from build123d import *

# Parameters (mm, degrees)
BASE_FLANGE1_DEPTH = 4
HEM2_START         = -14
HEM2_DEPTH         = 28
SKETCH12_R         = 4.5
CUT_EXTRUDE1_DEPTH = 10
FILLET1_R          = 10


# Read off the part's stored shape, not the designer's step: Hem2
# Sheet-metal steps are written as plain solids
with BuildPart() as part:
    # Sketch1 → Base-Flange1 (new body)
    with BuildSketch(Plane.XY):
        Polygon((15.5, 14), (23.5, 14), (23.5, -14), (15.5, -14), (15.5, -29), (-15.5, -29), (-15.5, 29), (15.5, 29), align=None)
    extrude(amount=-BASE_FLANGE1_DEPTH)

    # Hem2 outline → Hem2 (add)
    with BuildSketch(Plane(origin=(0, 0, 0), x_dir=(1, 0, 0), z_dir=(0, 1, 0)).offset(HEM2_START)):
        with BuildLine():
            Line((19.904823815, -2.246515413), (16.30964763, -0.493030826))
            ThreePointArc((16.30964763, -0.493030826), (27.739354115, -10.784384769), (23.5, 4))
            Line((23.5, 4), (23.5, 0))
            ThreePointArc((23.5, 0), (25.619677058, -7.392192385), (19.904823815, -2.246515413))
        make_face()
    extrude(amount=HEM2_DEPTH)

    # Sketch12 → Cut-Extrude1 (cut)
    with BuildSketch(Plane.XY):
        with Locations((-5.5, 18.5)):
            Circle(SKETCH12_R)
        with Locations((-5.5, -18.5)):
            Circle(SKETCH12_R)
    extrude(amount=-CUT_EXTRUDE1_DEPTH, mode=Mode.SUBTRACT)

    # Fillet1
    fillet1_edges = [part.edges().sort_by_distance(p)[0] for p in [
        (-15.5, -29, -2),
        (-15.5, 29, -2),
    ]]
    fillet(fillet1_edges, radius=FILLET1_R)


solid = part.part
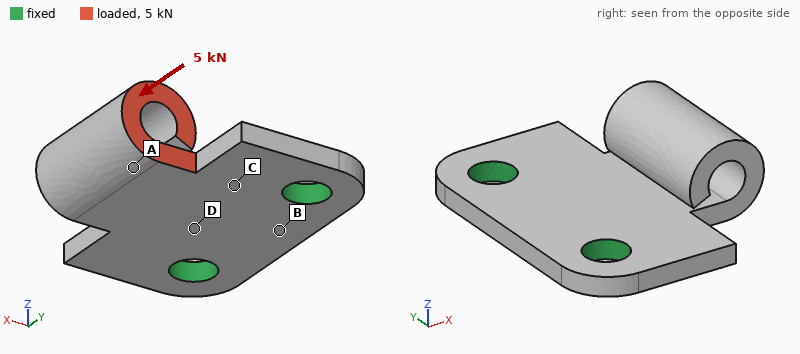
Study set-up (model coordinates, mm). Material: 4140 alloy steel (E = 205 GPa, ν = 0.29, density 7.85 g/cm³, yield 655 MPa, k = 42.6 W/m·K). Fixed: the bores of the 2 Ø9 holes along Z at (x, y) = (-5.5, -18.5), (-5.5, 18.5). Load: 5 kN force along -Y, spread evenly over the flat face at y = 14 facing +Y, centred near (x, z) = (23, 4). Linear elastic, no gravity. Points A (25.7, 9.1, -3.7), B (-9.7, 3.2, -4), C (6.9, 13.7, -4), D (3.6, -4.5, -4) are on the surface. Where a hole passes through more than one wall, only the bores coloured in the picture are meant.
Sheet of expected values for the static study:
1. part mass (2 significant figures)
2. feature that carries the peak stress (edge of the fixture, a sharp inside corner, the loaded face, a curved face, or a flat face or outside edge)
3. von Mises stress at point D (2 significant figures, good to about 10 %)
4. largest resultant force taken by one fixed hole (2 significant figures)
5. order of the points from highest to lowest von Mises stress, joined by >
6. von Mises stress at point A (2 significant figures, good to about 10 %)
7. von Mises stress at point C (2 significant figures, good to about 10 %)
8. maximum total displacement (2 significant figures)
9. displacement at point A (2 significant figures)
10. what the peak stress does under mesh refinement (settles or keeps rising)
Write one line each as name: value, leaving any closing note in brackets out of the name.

part mass: 85 g
feature that carries the peak stress: a sharp inside corner
von Mises stress at point D: 81 MPa
largest resultant force taken by one fixed hole: 4.2 kN
order of the points from highest to lowest von Mises stress, joined by >: A > C > D > B
von Mises stress at point A: 220 MPa
von Mises stress at point C: 150 MPa
maximum total displacement: 0.24 mm
displacement at point A: 0.086 mm
what the peak stress does under mesh refinement: keeps rising
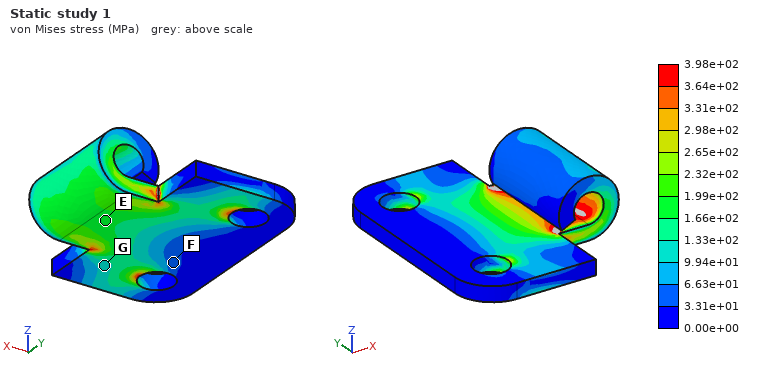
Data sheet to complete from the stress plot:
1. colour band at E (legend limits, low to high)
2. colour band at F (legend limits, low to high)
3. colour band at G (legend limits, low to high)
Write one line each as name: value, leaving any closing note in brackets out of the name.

colour band at E: 1.66e+02 to 1.99e+02 MPa
colour band at F: 3.31e+01 to 6.63e+01 MPa
colour band at G: 9.94e+01 to 1.33e+02 MPa
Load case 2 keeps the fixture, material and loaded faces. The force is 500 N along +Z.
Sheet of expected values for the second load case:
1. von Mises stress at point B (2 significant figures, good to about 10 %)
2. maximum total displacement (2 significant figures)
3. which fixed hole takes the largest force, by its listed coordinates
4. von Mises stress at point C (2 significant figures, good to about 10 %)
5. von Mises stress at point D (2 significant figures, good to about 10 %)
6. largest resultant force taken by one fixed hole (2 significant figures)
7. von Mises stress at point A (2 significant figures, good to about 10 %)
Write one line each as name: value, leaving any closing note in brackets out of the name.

von Mises stress at point B: 14 MPa
maximum total displacement: 0.13 mm
which fixed hole takes the largest force, by its listed coordinates: (-5.5, 18.5)
von Mises stress at point C: 77 MPa
von Mises stress at point D: 55 MPa
largest resultant force taken by one fixed hole: 460 N
von Mises stress at point A: 58 MPa
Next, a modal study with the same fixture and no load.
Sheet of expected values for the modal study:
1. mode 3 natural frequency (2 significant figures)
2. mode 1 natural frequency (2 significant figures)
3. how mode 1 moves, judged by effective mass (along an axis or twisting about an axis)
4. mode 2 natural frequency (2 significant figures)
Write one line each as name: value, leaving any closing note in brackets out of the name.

mode 3 natural frequency: 4700 Hz
mode 1 natural frequency: 2100 Hz
how mode 1 moves, judged by effective mass: along Z
mode 2 natural frequency: 4000 Hz
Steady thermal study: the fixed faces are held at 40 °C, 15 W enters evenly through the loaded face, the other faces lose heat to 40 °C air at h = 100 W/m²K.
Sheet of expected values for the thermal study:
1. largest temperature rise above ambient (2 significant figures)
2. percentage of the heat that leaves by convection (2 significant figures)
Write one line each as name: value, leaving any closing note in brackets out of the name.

largest temperature rise above ambient: 60 K
percentage of the heat that leaves by convection: 66 %
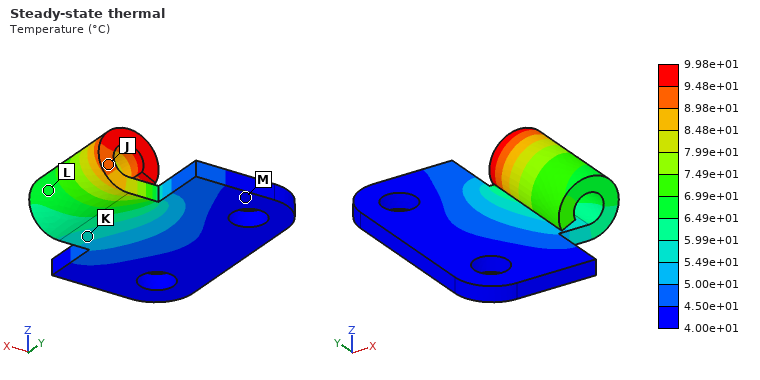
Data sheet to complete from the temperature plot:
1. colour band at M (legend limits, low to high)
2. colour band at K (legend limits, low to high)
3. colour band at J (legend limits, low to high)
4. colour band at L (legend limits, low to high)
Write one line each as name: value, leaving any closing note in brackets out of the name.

colour band at M: 4.00e+01 to 4.50e+01 °C
colour band at K: 5.49e+01 to 5.99e+01 °C
colour band at J: 8.98e+01 to 9.48e+01 °C
colour band at L: 6.49e+01 to 6.99e+01 °C
